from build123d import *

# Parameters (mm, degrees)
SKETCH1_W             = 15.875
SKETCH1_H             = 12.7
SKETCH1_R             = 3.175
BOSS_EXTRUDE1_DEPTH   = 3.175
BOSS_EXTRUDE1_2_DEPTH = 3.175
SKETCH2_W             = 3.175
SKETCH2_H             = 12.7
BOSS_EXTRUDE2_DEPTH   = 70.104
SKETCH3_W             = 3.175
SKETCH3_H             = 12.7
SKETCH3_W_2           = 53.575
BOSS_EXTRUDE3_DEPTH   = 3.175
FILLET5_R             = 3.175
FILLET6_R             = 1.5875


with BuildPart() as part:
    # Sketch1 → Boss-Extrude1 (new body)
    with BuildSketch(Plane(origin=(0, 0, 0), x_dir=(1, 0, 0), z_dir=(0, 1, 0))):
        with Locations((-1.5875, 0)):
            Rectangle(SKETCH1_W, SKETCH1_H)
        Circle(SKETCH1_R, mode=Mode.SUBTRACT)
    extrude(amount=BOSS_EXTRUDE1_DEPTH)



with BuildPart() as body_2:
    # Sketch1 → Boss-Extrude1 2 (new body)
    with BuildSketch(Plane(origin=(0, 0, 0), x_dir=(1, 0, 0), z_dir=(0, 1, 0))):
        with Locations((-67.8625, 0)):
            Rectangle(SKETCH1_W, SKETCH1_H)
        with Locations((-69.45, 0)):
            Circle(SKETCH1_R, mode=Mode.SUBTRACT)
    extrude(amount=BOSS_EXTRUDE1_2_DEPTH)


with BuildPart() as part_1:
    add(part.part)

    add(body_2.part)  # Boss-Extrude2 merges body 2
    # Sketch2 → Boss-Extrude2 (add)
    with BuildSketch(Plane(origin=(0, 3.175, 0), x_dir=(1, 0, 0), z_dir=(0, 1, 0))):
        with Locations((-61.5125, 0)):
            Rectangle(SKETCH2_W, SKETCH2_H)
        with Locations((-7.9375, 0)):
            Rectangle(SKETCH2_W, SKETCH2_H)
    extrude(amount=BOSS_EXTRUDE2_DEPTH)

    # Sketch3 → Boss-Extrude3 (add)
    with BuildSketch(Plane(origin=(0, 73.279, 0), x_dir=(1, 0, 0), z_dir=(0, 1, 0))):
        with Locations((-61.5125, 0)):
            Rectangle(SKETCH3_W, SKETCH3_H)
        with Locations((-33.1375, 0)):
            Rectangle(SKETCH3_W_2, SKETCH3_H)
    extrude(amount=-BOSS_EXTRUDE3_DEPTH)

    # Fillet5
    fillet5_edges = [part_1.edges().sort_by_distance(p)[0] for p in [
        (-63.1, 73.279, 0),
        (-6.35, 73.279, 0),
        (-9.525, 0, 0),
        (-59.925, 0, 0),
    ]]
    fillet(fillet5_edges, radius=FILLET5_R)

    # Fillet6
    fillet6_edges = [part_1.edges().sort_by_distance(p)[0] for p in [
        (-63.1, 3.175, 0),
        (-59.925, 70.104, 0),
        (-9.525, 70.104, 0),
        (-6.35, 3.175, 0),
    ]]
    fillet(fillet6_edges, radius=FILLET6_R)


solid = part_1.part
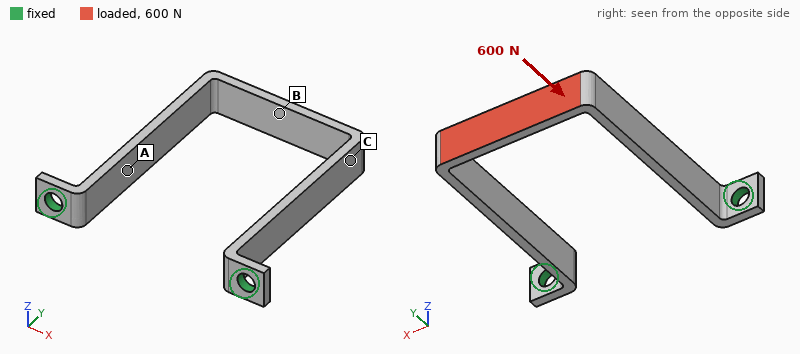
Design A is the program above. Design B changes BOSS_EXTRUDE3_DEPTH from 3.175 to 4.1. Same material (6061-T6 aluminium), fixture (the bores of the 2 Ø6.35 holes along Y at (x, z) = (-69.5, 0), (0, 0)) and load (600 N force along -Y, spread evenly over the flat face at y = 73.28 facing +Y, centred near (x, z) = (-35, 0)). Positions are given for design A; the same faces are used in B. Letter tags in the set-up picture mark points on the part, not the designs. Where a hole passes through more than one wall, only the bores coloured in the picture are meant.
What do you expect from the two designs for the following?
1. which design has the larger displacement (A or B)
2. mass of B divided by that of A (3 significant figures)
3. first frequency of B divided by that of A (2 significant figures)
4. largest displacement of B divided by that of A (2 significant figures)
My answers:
A
1.07
1.00
0.63
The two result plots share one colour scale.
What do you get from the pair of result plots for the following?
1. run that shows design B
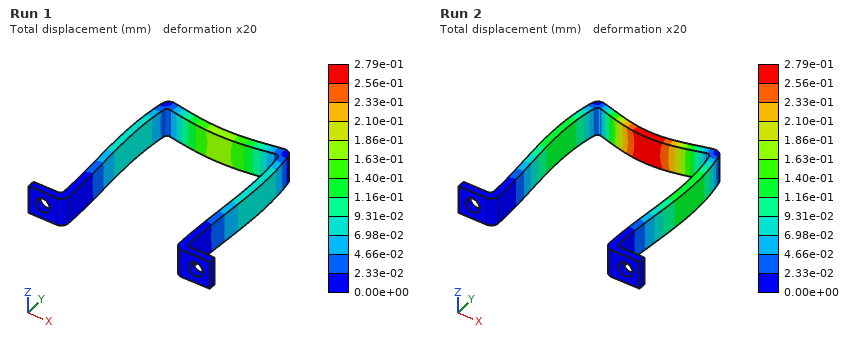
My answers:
Run 1
